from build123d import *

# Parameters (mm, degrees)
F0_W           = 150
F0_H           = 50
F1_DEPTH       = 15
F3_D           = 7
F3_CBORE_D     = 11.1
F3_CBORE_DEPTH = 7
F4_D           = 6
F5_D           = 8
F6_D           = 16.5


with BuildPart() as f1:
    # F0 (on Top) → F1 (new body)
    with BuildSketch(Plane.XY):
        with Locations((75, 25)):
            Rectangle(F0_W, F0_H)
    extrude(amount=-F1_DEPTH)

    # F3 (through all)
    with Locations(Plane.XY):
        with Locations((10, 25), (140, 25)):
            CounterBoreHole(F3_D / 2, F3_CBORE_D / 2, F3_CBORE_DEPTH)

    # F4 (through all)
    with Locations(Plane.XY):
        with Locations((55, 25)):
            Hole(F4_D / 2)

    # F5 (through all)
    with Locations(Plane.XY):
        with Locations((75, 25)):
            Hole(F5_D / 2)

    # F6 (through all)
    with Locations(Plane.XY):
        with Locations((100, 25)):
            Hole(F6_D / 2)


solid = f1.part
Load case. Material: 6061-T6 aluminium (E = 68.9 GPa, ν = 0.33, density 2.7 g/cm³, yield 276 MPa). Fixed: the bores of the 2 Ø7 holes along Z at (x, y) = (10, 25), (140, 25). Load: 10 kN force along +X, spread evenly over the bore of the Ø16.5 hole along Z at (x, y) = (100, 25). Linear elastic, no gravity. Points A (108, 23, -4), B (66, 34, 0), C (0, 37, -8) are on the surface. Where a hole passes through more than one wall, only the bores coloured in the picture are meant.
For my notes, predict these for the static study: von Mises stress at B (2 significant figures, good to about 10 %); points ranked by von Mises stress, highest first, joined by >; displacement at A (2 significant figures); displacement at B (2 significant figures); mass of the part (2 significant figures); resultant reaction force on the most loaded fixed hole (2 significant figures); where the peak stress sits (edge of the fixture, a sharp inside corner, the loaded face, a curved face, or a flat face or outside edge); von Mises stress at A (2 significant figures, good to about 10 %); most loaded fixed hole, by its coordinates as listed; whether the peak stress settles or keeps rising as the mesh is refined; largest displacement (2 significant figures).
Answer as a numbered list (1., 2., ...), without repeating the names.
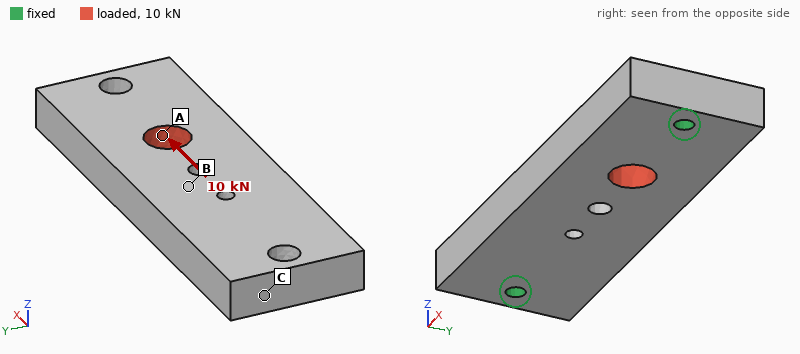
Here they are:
1. 8.5 MPa
2. A > B > C
3. 12 µm
4. 7.0 µm
5. 290 g
6. 6.1 kN
7. edge of the fixture
8. 16 MPa
9. (140, 25)
10. keeps rising
11. 14 µm
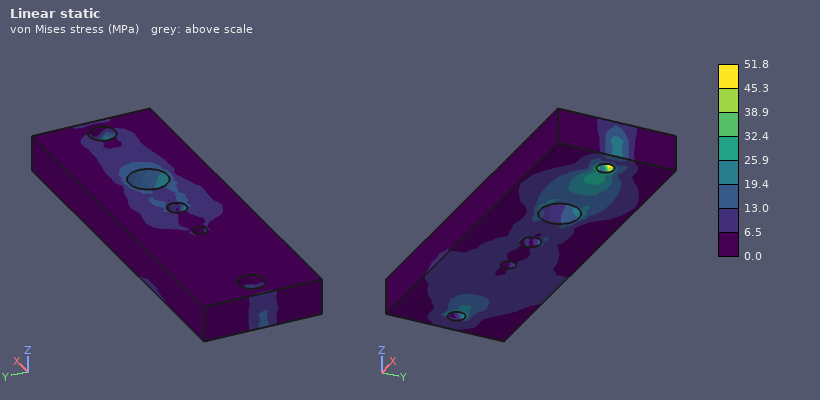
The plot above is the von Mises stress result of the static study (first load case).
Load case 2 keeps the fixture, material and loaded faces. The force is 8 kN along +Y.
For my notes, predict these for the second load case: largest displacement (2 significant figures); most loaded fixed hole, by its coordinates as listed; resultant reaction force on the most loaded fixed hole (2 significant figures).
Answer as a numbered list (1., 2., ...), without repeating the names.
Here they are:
1. 46 µm
2. (140, 25)
3. 5.6 kN
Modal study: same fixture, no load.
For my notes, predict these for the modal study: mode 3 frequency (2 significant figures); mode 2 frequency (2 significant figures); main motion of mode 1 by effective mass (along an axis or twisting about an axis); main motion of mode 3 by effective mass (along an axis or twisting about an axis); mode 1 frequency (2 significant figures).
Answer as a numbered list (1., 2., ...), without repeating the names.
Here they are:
1. 5900 Hz
2. 3800 Hz
3. along Z
4. along Y
5. 3000 Hz
